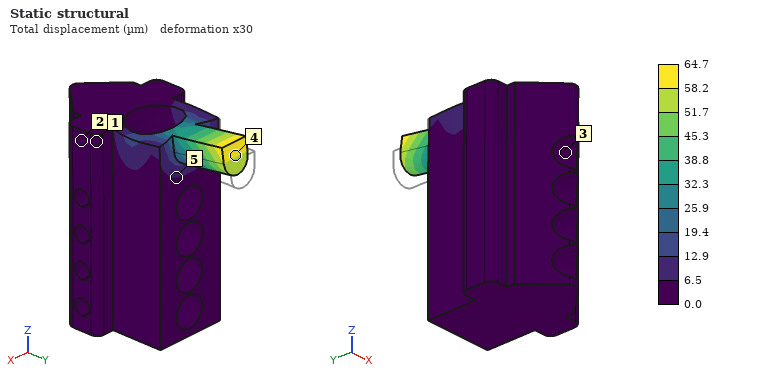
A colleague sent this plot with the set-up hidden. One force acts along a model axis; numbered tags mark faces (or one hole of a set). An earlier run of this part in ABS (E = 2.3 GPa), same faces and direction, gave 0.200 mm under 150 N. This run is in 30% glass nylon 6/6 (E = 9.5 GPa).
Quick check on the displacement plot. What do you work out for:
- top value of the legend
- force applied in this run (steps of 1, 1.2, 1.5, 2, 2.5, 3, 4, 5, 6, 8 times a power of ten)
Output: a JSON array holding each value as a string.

["64.7 µm", "200 N"]
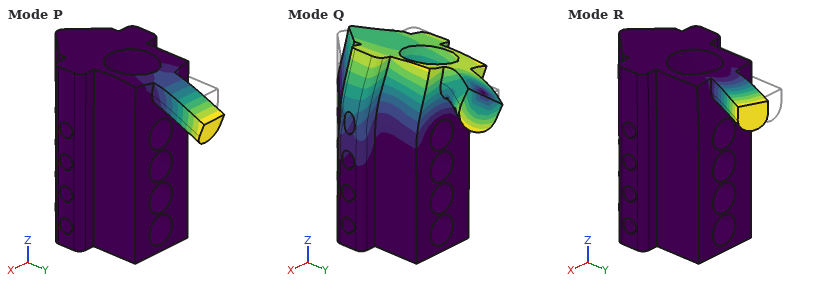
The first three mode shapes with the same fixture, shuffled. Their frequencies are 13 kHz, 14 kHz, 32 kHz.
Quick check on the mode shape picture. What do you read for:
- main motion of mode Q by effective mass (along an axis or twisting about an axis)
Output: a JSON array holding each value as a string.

["along X"]
